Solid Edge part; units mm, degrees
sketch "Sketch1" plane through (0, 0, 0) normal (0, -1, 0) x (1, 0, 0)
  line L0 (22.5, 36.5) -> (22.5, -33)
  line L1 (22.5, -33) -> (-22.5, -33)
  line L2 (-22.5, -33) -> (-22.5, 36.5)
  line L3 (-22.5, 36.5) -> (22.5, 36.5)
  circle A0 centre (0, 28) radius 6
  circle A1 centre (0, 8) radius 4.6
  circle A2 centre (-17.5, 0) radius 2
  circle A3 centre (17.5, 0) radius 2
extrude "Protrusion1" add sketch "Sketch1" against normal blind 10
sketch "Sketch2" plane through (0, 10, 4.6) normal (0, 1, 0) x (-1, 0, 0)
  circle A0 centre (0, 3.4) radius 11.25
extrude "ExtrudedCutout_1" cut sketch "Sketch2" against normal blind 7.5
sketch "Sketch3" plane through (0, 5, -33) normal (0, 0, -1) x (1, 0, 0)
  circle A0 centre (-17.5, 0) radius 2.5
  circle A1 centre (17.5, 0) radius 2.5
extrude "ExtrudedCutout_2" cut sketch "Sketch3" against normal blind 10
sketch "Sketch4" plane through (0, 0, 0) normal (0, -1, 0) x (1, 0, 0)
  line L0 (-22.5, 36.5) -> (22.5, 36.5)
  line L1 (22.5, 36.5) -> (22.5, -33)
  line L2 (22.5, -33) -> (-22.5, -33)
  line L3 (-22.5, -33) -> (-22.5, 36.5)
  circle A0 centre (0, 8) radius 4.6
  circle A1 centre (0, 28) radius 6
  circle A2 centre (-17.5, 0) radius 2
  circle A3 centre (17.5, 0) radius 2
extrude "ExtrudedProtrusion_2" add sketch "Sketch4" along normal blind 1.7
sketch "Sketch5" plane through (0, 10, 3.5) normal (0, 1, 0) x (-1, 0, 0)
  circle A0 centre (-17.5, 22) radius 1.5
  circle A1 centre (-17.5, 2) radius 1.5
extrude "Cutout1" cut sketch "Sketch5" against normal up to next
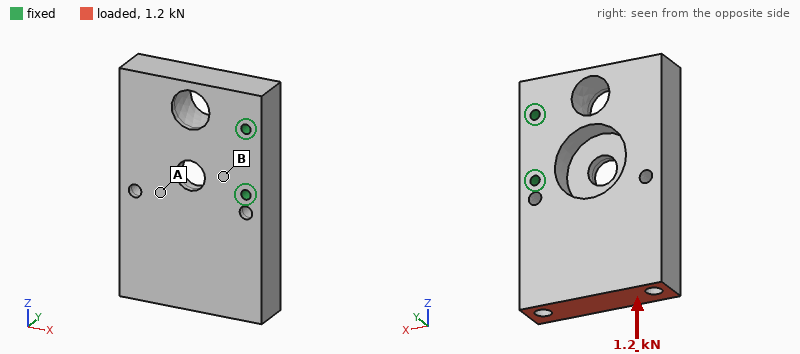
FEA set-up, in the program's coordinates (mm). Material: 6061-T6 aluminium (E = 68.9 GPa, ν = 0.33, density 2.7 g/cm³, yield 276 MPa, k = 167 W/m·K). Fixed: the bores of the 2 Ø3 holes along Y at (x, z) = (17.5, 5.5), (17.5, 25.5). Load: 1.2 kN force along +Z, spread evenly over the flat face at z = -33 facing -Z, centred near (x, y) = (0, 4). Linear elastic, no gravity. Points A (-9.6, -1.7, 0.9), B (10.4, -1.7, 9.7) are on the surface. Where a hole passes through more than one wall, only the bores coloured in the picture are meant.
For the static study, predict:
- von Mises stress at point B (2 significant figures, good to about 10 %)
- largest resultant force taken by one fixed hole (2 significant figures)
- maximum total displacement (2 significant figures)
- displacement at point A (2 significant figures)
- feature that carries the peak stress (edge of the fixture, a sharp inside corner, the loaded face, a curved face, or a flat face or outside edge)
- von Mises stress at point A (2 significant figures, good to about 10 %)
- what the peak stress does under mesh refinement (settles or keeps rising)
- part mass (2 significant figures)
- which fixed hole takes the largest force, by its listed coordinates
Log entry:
14 MPa
1.2 kN
24 µm
11 µm
edge of the fixture
4.3 MPa
keeps rising
84 g
(17.5, 5.5)
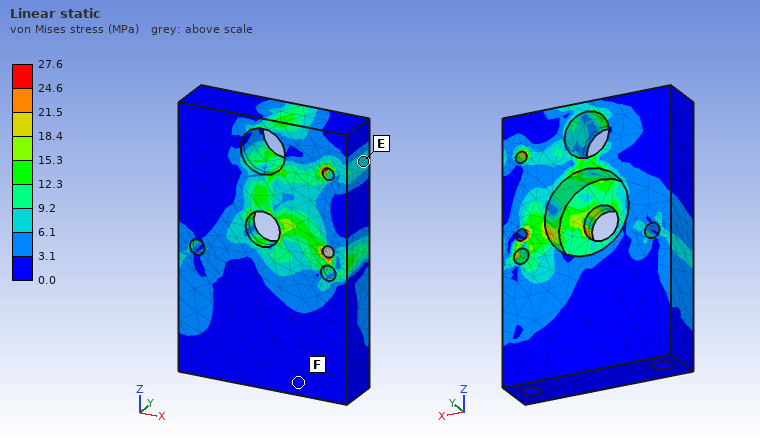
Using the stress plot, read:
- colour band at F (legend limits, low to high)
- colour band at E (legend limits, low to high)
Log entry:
0.0 to 3.1 MPa
6.1 to 9.2 MPa
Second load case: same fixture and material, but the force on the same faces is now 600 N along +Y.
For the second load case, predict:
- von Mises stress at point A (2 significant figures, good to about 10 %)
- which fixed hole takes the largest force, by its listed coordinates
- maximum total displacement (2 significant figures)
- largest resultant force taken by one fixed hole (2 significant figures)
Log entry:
17 MPa
(17.5, 5.5)
0.12 mm
1.0 kN
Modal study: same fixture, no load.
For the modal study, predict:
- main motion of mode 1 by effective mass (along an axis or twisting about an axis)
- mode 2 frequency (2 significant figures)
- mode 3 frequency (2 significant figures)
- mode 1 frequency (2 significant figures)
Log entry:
along Y
4000 Hz
4600 Hz
2600 Hz
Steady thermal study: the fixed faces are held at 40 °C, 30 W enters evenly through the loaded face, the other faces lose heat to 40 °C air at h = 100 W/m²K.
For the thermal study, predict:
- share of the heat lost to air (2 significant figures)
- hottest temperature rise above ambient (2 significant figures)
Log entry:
26 %
19 K
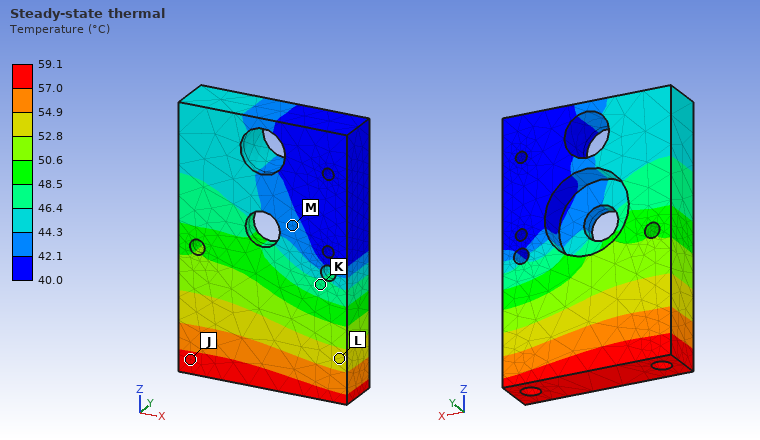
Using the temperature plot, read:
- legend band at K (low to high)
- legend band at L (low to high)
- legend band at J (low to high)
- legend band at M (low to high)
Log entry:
46.4 to 48.5 °C
52.8 to 54.9 °C
57.0 to 59.1 °C
42.1 to 44.3 °C
